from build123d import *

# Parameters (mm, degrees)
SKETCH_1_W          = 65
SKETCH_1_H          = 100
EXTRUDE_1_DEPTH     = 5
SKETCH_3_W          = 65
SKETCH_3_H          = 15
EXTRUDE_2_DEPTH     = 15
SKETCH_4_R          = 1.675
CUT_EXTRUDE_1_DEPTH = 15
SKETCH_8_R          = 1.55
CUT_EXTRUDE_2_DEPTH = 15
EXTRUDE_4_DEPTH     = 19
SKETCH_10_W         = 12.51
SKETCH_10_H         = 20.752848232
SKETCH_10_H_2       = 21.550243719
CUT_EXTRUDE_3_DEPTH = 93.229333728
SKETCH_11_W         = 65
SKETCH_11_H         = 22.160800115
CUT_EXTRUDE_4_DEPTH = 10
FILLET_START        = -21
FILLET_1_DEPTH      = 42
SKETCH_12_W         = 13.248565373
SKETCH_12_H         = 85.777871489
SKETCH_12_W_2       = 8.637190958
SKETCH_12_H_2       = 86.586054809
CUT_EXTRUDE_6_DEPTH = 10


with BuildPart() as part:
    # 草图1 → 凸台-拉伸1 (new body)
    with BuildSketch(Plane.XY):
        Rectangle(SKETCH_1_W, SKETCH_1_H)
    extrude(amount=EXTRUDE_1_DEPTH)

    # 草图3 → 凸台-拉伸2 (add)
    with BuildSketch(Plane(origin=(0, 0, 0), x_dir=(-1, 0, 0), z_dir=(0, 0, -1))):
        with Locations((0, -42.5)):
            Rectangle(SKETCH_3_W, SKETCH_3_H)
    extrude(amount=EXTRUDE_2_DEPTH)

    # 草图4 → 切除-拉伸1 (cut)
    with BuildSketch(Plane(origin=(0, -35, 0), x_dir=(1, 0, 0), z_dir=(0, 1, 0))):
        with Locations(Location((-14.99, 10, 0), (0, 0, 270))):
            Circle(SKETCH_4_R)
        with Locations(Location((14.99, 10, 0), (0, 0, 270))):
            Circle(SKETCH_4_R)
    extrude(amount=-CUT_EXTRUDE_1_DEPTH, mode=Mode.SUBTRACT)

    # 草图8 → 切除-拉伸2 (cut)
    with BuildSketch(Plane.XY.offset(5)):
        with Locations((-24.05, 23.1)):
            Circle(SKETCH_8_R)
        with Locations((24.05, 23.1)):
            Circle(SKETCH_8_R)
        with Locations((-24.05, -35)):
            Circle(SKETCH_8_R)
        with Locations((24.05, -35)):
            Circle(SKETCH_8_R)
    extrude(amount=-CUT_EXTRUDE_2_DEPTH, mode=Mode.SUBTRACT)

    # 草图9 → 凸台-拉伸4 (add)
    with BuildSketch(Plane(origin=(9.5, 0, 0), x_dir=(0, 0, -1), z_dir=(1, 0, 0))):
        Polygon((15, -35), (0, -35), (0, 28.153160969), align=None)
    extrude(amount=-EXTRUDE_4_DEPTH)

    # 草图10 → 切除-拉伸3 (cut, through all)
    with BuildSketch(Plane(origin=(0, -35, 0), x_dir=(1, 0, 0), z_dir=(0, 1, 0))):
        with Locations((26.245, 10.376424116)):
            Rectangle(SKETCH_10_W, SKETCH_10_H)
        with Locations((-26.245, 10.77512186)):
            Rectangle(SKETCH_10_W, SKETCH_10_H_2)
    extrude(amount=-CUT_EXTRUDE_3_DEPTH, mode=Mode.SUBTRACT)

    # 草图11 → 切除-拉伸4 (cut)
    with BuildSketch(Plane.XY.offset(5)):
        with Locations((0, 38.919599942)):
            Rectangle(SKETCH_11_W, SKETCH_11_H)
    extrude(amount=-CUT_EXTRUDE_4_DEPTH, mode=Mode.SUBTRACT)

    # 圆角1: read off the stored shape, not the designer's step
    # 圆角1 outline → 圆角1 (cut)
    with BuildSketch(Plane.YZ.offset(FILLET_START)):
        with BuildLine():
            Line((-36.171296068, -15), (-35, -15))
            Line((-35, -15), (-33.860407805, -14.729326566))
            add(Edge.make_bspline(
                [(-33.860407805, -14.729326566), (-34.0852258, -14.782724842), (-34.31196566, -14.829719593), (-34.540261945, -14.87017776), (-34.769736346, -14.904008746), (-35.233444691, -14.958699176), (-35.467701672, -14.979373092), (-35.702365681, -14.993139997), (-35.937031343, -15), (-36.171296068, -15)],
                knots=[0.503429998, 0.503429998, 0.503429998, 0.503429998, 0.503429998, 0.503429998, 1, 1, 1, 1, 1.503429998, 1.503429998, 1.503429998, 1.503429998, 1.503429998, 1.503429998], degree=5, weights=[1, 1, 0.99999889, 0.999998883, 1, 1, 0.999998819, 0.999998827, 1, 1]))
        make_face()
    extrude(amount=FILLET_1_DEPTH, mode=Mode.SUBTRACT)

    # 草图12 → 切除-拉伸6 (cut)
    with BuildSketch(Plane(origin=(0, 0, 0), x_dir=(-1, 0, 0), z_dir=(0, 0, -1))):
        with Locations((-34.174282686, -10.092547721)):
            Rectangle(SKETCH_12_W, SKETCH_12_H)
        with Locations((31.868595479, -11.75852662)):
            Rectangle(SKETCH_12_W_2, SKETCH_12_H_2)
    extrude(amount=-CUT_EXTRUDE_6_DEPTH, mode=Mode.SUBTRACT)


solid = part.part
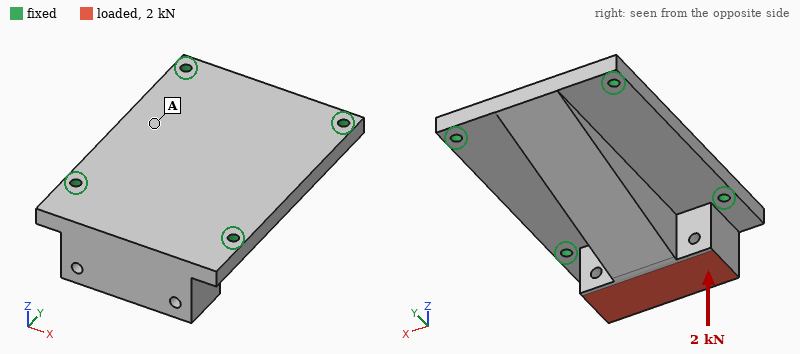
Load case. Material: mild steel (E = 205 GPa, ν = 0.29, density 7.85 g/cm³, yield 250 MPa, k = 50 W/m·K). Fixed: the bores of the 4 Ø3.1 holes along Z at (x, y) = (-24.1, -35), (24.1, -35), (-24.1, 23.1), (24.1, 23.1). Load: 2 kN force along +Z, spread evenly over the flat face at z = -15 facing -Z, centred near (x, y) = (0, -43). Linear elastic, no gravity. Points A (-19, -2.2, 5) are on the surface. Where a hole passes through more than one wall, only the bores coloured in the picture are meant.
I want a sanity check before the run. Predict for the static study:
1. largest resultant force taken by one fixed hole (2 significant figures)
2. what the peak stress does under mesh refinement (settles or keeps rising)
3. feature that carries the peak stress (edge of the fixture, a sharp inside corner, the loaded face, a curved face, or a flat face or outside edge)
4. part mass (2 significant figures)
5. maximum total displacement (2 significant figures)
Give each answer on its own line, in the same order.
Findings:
1.2 kN
keeps rising
edge of the fixture
310 g
8.7 µm
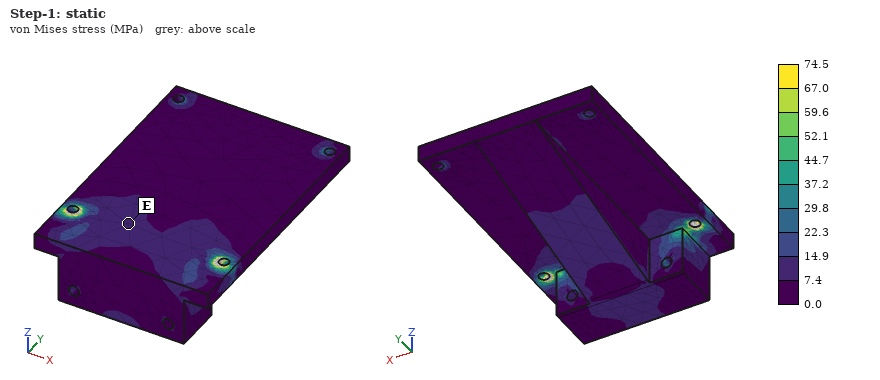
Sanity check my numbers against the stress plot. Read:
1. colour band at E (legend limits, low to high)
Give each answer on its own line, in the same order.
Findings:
7.4 to 14.9 MPa
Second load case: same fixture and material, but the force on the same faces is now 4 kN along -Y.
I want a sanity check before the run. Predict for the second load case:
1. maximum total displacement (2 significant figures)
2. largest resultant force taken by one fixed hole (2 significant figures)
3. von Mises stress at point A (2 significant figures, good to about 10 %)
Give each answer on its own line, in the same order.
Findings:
21 µm
1.3 kN
16 MPa
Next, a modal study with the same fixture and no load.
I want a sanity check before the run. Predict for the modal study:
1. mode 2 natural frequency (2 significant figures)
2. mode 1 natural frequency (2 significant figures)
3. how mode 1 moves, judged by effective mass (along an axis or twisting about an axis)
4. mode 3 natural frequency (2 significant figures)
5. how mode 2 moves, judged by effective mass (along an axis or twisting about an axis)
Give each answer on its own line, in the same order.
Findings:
8300 Hz
5900 Hz
along Z
11 kHz
along Z
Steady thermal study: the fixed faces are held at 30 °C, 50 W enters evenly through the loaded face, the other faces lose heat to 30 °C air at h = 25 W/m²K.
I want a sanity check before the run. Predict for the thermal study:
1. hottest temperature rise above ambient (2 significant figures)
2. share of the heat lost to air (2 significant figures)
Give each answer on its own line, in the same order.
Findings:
66 K
15 %
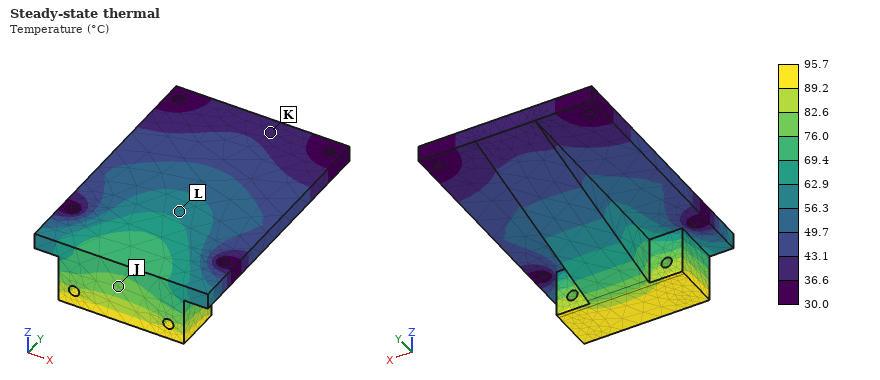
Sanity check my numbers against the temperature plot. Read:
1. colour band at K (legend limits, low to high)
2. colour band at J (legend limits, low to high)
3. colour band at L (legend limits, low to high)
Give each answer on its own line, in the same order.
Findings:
36.6 to 43.1 °C
76.0 to 82.6 °C
56.3 to 62.9 °C
